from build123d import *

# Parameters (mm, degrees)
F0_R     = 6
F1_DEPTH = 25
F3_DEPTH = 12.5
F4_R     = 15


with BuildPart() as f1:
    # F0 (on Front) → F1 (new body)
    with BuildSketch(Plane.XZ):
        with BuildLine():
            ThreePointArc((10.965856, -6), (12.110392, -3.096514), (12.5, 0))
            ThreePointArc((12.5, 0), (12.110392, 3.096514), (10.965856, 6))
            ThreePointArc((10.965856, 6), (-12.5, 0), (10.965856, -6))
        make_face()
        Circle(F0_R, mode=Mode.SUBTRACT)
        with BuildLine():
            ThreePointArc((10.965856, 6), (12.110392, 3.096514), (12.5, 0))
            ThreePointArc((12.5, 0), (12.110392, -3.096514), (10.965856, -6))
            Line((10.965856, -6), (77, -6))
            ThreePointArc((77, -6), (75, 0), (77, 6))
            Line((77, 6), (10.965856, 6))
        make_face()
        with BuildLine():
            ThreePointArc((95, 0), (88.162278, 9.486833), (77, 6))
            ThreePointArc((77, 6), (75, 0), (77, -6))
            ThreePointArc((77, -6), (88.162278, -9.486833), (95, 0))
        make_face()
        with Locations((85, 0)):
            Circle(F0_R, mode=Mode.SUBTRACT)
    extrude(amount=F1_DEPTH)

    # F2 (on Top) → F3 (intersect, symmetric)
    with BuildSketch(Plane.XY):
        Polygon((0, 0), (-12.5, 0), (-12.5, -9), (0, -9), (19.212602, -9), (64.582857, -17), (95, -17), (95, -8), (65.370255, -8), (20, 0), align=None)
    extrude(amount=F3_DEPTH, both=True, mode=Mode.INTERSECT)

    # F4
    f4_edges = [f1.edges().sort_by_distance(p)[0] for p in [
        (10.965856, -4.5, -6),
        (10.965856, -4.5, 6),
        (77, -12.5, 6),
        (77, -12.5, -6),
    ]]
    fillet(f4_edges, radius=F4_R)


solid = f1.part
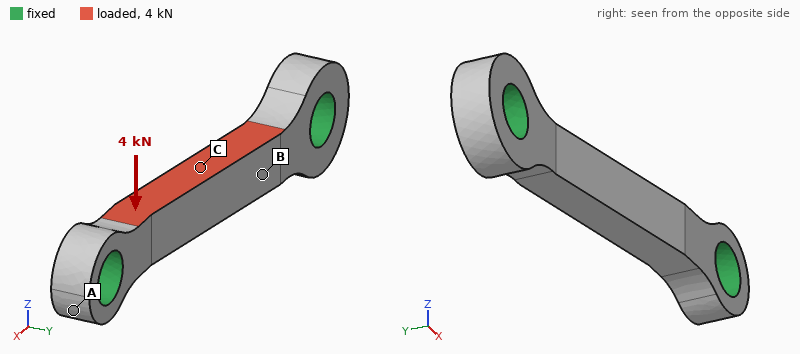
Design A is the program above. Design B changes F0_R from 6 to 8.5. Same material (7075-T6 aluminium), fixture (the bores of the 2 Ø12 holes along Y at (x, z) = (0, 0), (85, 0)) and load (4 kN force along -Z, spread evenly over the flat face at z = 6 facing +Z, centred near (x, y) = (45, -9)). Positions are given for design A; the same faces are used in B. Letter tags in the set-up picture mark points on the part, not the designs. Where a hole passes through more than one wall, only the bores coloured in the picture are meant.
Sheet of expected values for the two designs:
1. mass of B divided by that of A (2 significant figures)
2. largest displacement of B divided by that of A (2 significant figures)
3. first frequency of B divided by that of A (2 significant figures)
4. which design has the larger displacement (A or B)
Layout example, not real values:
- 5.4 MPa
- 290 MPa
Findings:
- 0.83
- 0.84
- 1.1
- A
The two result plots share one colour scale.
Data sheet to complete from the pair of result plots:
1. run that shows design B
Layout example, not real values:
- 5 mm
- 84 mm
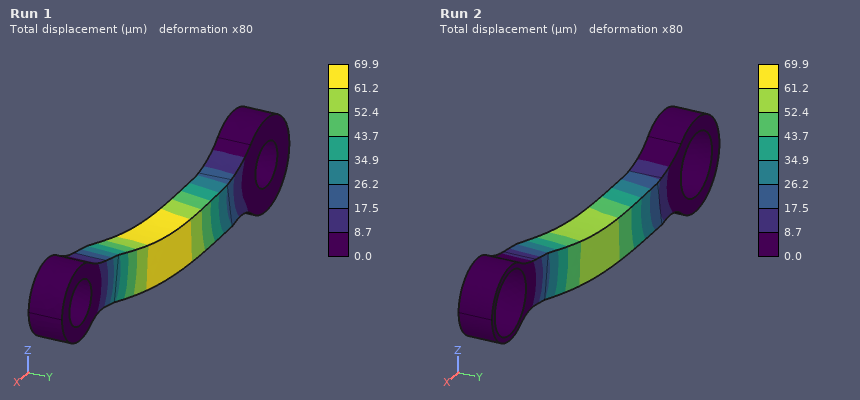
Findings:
- Run 2
